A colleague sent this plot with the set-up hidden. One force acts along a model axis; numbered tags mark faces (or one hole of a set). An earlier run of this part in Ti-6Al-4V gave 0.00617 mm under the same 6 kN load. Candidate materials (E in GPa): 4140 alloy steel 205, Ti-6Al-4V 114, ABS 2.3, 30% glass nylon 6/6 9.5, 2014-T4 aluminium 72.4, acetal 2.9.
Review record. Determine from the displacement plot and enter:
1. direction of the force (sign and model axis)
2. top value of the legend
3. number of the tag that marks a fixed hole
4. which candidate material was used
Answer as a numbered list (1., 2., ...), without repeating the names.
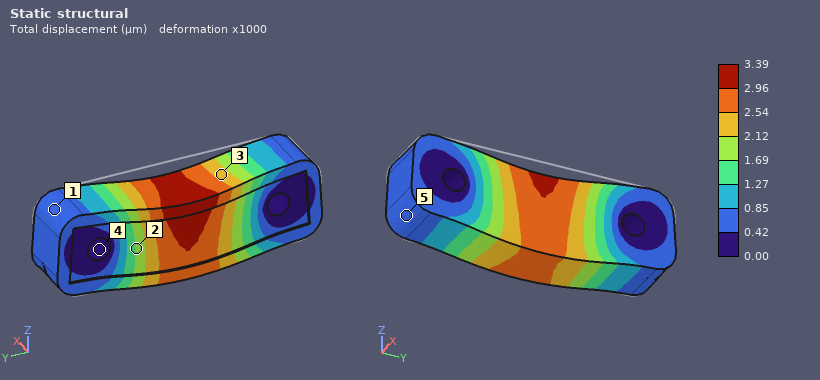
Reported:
1. -Z
2. 3.39 µm
3. 4
4. 4140 alloy steel
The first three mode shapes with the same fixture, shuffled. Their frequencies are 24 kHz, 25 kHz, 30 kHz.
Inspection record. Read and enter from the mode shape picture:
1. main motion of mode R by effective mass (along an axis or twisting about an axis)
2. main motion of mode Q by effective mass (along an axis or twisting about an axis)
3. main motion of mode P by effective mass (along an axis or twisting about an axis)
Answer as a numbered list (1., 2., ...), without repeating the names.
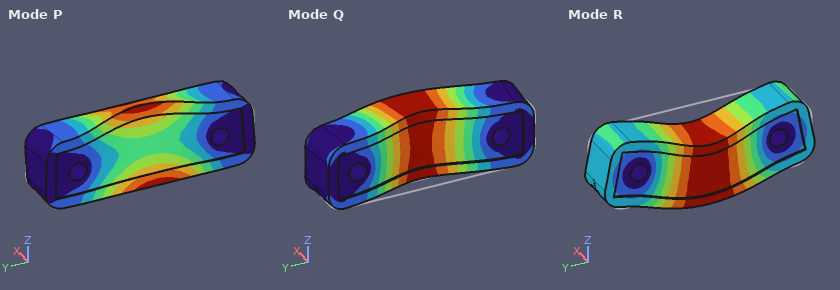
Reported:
1. along Z
2. along X
3. twisting about Y
